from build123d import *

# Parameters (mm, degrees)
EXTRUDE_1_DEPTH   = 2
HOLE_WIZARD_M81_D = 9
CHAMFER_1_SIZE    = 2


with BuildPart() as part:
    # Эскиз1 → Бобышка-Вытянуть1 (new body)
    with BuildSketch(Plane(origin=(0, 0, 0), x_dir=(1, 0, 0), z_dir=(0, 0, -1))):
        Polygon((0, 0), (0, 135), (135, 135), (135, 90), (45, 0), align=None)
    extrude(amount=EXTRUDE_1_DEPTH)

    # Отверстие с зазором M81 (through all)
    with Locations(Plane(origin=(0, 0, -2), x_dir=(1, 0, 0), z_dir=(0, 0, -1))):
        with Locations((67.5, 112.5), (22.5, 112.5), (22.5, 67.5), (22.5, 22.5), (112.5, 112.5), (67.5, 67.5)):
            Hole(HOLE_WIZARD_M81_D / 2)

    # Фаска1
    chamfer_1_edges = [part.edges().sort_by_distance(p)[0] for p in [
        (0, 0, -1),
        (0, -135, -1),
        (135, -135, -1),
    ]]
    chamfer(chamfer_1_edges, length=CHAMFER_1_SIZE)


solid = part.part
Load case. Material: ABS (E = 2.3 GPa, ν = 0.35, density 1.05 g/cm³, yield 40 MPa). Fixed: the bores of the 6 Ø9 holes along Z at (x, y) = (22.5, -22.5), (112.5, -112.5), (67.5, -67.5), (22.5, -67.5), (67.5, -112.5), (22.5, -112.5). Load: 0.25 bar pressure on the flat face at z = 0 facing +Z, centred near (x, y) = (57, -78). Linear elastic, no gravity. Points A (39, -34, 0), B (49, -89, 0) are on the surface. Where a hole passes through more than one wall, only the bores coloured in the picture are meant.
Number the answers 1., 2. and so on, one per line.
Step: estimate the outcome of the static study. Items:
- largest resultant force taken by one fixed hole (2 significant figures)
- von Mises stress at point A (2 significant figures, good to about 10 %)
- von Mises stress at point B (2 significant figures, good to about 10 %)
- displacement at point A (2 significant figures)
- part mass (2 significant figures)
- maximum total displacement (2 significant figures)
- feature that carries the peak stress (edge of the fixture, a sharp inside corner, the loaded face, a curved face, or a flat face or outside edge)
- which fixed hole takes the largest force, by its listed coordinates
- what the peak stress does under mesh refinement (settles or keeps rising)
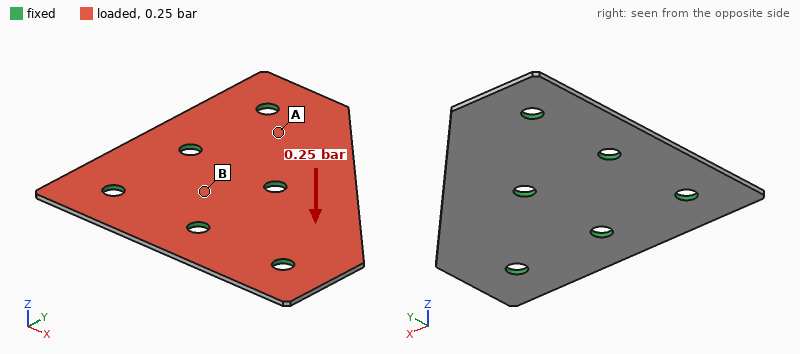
1. 80 N
2. 6.4 MPa
3. 1.9 MPa
4. 0.41 mm
5. 29 g
6. 2.3 mm
7. edge of the fixture
8. (67.5, -67.5)
9. keeps rising
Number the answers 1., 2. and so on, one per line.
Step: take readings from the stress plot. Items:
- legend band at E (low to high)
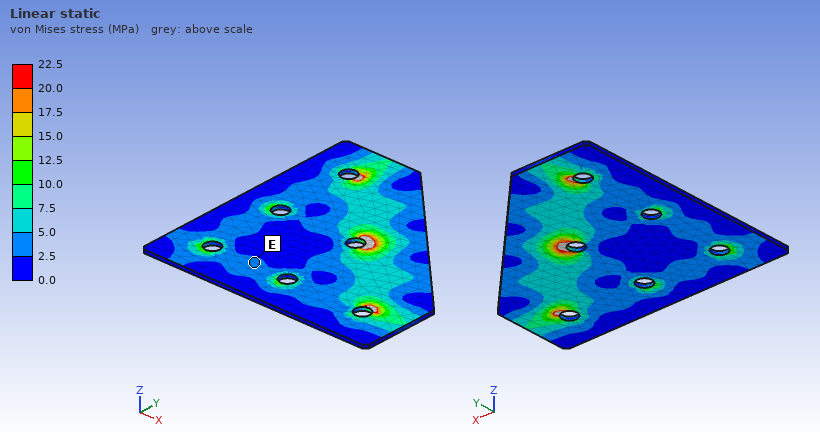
1. 2.5 to 5.0 MPa
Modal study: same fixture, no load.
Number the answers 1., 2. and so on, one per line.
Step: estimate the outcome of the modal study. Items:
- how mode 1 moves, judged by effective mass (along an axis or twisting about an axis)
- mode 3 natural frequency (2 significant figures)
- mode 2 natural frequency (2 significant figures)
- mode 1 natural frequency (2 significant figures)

1. along Z
2. 860 Hz
3. 530 Hz
4. 470 Hz
